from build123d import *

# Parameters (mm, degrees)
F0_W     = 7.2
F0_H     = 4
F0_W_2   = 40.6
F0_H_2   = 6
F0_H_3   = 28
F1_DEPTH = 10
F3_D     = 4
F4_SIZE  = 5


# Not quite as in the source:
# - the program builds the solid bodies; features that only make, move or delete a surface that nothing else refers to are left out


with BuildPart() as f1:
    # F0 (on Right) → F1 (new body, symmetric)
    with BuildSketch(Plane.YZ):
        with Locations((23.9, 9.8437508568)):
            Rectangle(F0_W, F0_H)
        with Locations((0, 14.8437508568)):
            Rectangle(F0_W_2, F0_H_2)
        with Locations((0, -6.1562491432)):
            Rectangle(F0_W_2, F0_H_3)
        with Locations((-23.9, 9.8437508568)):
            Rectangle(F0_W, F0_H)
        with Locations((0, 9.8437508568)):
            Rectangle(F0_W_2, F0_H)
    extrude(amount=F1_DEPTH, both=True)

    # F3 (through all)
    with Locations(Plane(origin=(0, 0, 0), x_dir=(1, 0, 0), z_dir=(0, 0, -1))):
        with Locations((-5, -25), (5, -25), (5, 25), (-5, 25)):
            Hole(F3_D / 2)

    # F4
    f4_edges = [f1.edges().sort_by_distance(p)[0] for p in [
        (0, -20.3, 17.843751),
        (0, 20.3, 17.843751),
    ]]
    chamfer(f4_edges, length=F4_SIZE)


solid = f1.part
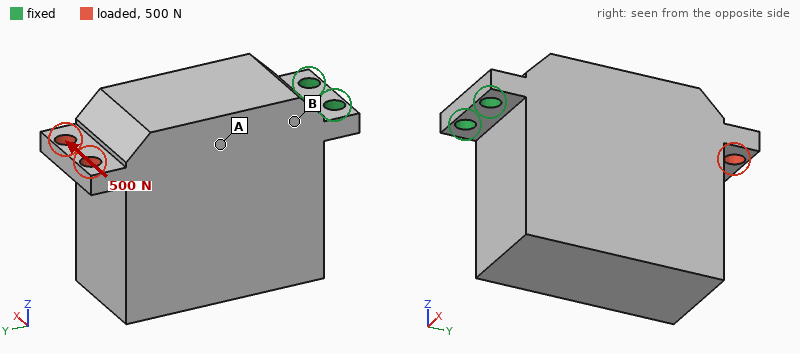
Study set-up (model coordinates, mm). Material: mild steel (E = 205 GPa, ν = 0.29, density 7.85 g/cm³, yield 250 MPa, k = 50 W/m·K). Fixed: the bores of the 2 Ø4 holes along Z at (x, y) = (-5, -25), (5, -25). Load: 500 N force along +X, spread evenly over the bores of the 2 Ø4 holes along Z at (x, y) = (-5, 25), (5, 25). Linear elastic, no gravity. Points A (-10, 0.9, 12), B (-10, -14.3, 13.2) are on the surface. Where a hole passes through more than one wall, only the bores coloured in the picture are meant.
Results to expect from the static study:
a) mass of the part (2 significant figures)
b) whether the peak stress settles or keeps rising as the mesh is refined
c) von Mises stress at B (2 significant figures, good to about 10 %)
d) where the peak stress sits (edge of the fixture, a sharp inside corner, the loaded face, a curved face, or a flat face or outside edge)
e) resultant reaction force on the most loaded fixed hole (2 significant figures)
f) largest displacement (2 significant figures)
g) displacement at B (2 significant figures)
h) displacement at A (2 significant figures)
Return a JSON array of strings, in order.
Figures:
["250 g", "keeps rising", "23 MPa", "edge of the fixture", "2.0 kN", "26 µm", "5.0 µm", "11 µm"]
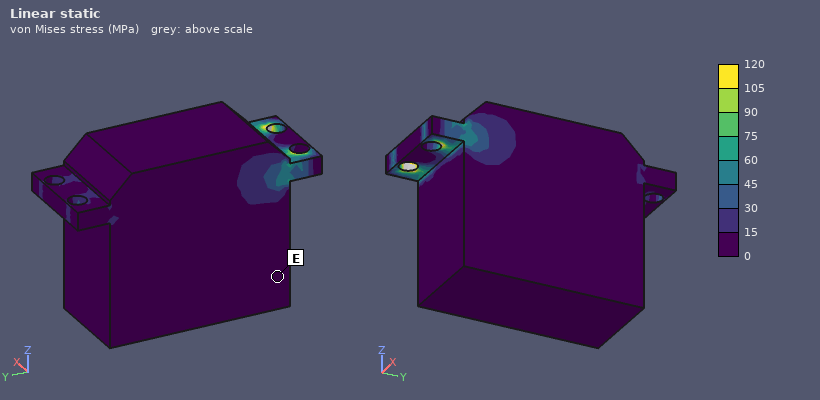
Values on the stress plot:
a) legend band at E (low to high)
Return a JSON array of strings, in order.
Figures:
["0 to 15 MPa"]
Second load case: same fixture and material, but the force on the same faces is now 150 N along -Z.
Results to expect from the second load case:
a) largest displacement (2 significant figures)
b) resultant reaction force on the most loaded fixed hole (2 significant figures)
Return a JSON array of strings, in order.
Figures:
["83 µm", "75 N"]
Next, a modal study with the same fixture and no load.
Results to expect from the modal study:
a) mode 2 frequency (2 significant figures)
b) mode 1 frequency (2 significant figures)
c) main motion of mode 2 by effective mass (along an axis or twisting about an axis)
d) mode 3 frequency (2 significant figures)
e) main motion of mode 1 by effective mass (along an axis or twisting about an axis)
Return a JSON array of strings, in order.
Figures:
["2300 Hz", "730 Hz", "along X", "4300 Hz", "along Z"]
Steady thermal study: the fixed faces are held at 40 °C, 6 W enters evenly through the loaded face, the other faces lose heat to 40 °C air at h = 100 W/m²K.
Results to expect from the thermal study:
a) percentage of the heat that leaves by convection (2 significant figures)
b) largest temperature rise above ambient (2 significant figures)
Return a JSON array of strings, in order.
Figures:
["63 %", "23 K"]
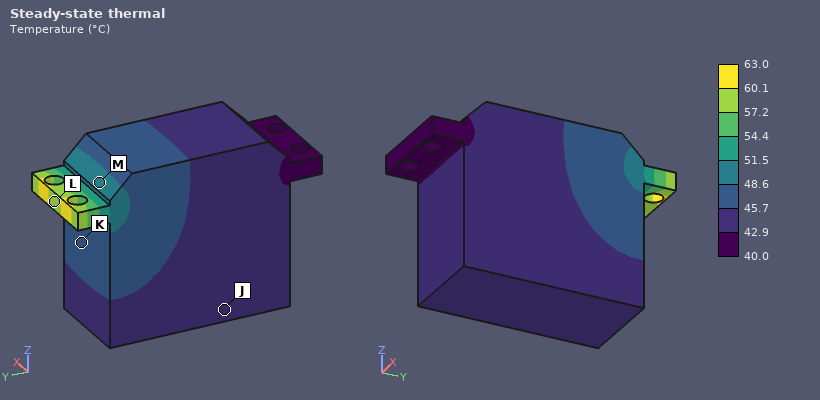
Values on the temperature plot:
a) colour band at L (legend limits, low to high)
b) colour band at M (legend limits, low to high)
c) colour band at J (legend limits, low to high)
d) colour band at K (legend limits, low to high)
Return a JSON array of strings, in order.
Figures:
["57.2 to 60.1 °C", "48.6 to 51.5 °C", "42.9 to 45.7 °C", "45.7 to 48.6 °C"]
